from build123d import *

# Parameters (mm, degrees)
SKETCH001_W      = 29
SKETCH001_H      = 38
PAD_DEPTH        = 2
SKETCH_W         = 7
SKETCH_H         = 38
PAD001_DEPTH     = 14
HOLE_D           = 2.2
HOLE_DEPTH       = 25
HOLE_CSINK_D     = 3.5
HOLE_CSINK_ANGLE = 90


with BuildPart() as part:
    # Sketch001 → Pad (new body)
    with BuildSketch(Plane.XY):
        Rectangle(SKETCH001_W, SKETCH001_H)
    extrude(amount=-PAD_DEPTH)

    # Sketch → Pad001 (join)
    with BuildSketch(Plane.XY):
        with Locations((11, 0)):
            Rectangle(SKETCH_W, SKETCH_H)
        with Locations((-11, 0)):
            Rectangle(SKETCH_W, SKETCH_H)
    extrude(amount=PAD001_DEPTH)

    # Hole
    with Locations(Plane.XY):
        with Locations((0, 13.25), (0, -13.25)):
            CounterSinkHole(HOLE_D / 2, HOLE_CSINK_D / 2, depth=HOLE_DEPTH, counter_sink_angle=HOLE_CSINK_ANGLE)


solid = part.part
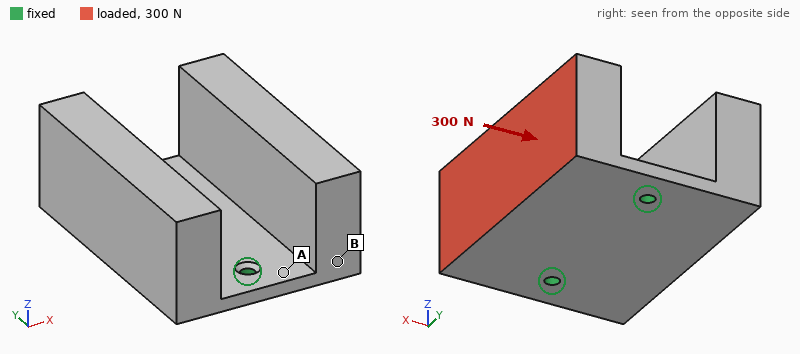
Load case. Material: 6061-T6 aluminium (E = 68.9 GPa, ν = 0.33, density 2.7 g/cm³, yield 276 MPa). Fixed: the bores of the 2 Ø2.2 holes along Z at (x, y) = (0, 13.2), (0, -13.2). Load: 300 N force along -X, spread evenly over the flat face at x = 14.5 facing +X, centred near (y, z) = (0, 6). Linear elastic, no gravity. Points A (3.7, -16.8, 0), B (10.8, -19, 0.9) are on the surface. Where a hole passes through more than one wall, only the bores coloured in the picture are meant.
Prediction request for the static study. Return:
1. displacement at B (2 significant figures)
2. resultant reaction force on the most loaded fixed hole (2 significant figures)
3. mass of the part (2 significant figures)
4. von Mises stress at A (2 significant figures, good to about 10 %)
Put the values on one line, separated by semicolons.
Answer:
0.099 mm; 150 N; 26 g; 87 MPa
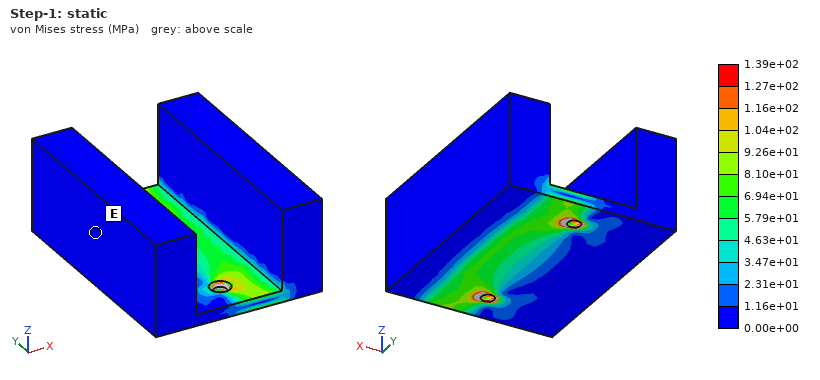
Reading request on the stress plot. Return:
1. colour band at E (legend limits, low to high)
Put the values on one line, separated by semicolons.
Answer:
0.00e+00 to 1.16e+01 MPa
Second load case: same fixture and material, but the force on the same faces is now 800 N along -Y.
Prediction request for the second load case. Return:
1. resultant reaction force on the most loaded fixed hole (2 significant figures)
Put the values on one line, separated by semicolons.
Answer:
620 N
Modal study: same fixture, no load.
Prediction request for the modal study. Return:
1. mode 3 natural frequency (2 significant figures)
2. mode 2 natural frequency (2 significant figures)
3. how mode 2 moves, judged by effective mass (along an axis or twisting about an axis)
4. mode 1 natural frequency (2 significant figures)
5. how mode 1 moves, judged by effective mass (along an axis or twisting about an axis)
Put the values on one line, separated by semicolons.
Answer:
5000 Hz; 2000 Hz; along Z; 1400 Hz; along X
